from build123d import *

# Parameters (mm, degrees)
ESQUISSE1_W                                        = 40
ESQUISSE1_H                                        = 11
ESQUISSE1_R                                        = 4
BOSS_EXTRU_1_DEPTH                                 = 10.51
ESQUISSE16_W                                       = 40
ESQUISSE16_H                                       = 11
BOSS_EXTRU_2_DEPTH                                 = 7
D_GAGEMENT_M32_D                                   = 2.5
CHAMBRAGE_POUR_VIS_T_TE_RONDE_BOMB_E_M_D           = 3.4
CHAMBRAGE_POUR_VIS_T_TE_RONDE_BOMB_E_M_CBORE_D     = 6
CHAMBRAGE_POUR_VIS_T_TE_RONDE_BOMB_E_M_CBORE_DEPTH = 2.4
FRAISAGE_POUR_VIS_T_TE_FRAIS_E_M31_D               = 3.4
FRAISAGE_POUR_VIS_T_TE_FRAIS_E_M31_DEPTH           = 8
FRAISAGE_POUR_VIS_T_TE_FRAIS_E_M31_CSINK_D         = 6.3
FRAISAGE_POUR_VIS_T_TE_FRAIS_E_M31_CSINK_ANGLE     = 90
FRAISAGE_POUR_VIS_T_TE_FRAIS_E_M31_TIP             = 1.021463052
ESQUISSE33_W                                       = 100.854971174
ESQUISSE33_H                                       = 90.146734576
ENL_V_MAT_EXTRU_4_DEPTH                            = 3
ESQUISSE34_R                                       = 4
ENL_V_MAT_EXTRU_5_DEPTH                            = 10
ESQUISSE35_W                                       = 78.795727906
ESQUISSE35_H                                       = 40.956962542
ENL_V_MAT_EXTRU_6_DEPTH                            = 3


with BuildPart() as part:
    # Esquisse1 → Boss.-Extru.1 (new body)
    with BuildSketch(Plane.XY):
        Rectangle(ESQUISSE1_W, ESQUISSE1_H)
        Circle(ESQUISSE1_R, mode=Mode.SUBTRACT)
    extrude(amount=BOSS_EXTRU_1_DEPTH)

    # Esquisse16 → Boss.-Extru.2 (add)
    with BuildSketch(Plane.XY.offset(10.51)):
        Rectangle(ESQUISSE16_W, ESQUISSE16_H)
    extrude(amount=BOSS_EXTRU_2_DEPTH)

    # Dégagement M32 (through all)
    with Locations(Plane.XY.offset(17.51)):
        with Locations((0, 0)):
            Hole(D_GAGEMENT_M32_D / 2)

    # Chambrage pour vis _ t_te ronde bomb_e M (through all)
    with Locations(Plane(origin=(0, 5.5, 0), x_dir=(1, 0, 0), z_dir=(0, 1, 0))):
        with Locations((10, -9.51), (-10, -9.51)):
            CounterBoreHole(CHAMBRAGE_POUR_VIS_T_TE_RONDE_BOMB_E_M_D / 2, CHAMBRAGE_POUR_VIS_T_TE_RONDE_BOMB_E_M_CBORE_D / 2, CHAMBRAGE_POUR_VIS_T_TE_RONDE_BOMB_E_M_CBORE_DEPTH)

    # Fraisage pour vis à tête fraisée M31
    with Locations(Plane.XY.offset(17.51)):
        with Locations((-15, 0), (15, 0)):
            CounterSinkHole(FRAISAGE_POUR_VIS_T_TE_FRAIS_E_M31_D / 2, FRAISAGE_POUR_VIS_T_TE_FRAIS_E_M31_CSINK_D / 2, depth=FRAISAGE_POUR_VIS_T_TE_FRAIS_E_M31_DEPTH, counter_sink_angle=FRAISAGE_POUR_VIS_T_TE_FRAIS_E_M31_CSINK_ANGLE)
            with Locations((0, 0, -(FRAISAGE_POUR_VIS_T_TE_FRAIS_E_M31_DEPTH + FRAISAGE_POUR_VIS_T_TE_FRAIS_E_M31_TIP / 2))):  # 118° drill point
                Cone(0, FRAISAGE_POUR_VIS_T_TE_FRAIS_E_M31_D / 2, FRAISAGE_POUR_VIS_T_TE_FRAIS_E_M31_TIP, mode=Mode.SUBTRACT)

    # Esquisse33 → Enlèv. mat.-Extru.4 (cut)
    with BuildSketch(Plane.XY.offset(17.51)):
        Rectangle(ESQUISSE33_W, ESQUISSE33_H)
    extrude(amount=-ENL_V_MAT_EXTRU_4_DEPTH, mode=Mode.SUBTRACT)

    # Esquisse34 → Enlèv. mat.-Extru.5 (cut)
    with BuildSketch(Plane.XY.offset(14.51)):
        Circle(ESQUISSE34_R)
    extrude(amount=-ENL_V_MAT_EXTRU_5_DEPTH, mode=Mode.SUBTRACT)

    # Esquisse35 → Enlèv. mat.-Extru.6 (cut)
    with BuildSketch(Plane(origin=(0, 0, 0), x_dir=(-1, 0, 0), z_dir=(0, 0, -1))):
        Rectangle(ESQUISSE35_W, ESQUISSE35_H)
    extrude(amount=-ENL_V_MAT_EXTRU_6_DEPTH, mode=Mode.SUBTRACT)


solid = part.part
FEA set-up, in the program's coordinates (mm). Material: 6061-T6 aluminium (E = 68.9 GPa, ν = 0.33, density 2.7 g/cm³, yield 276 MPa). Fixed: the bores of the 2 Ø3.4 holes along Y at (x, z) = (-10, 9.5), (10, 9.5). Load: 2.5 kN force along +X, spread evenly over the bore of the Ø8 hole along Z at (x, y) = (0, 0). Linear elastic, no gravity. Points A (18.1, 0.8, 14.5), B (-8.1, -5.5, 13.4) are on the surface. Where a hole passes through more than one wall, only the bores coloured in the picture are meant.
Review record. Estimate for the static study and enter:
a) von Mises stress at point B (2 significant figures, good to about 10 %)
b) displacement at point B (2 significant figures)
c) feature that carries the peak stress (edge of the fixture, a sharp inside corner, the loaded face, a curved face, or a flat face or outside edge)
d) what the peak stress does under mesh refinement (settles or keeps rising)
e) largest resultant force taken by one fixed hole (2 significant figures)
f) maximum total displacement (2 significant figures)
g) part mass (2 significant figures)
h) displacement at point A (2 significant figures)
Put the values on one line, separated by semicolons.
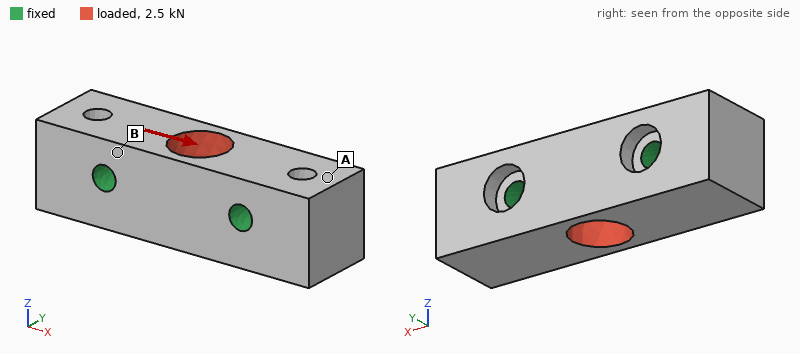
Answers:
6.9 MPa; 0.46 µm; edge of the fixture; keeps rising; 1.3 kN; 2.6 µm; 11 g; 0.71 µm
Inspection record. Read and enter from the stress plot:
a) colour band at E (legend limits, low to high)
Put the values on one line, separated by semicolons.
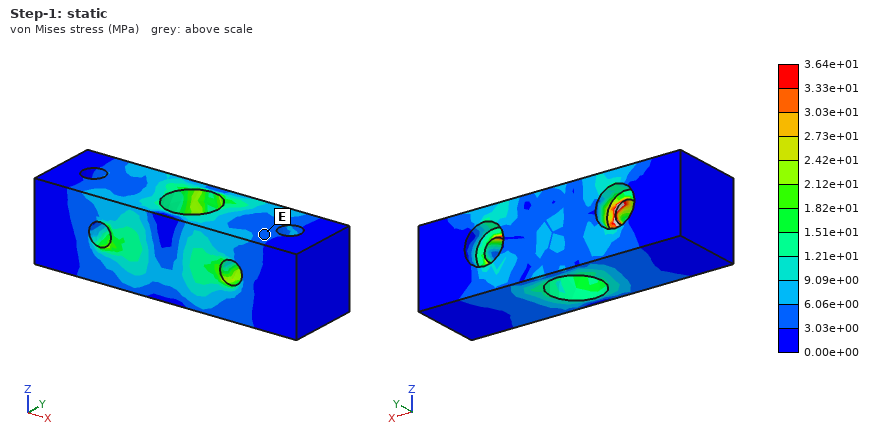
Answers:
3.03e+00 to 6.06e+00 MPa
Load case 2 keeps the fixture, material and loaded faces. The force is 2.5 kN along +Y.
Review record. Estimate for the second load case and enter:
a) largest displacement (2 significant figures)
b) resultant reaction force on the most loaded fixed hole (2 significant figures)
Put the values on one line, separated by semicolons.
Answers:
8.0 µm; 1.3 kN
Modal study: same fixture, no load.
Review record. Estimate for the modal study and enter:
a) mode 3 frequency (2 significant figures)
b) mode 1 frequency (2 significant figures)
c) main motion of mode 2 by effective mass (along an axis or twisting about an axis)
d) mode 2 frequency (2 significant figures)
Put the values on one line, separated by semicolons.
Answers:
42 kHz; 36 kHz; twisting about Y; 39 kHz
